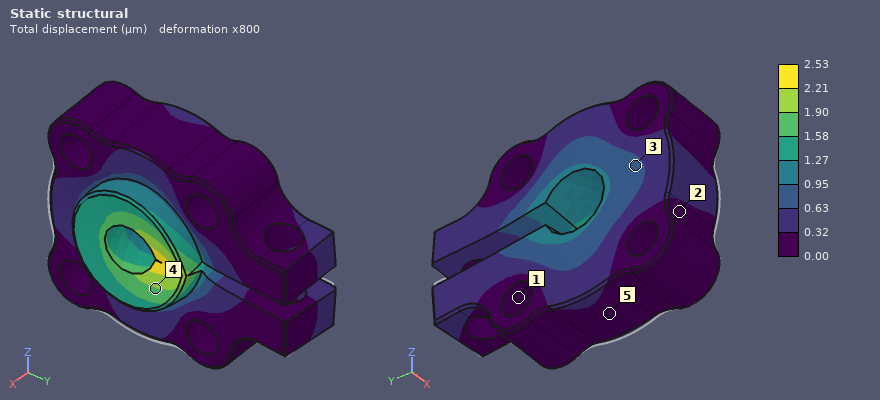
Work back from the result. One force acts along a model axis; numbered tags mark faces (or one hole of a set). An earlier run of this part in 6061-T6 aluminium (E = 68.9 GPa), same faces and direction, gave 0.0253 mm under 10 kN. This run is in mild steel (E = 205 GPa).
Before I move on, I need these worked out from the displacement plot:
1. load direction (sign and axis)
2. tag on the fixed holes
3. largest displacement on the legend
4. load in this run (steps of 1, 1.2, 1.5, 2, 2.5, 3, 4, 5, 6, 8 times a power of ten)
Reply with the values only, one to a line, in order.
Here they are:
-X
1
2.53 µm
3 kN
